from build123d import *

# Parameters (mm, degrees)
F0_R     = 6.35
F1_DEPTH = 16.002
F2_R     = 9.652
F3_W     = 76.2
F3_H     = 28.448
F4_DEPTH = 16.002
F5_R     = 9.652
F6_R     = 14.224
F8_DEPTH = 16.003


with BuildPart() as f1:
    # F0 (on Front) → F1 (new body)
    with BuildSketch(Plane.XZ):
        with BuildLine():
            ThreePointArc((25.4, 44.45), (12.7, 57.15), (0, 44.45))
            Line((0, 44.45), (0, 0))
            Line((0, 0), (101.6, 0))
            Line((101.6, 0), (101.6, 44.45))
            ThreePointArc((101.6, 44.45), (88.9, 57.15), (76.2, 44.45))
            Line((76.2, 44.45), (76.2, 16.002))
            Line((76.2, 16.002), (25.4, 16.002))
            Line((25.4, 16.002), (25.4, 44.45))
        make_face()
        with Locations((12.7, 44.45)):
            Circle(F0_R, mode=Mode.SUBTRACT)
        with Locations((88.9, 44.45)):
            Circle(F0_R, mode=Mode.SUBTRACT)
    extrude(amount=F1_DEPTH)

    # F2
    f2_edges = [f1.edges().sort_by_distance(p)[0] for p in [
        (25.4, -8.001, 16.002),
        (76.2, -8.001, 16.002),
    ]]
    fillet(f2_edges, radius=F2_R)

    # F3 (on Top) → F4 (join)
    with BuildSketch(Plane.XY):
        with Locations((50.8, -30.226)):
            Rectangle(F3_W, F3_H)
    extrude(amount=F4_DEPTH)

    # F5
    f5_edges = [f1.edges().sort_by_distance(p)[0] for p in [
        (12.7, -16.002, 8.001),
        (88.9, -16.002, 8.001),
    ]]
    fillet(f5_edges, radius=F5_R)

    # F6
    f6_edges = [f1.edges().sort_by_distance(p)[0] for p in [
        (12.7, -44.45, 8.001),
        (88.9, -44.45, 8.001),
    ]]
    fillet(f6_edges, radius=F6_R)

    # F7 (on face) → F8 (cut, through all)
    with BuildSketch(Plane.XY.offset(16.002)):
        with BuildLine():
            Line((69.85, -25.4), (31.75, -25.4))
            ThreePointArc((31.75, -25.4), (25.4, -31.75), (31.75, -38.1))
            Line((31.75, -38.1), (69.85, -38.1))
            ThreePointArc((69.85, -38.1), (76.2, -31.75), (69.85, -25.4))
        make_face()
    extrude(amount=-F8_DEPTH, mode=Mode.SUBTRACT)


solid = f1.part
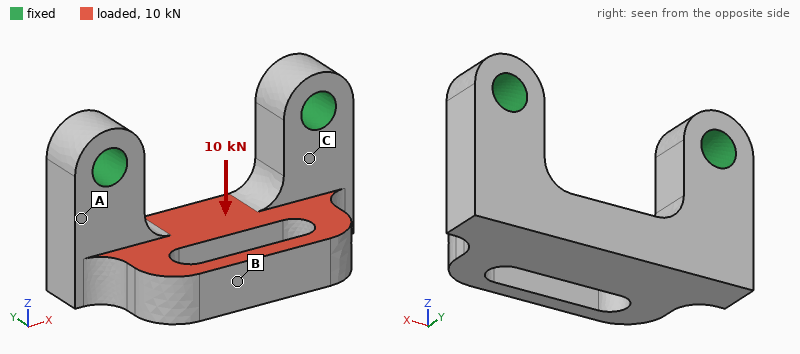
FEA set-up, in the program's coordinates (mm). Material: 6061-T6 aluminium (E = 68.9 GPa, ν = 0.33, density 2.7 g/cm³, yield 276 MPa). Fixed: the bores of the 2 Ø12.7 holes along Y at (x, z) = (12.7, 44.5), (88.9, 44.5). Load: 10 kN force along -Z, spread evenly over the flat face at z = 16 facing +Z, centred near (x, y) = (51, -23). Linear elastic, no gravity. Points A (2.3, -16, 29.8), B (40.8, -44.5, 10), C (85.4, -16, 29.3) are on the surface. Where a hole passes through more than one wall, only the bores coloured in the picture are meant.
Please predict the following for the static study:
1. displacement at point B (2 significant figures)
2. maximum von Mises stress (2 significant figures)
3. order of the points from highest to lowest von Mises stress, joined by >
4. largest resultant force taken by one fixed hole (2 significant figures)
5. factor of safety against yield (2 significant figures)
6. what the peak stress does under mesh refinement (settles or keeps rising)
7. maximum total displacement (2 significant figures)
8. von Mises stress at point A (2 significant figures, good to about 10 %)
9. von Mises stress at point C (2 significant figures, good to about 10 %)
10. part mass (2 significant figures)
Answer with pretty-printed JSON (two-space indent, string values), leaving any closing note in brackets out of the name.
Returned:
{
  "displacement at point B": "0.22 mm",
  "maximum von Mises stress": "150 MPa",
  "order of the points from highest to lowest von Mises stress, joined by >": "C > A > B",
  "largest resultant force taken by one fixed hole": "5.4 kN",
  "factor of safety against yield": "1.8",
  "what the peak stress does under mesh refinement": "settles",
  "maximum total displacement": "0.25 mm",
  "von Mises stress at point A": "61 MPa",
  "von Mises stress at point C": "93 MPa",
  "part mass": "210 g"
}
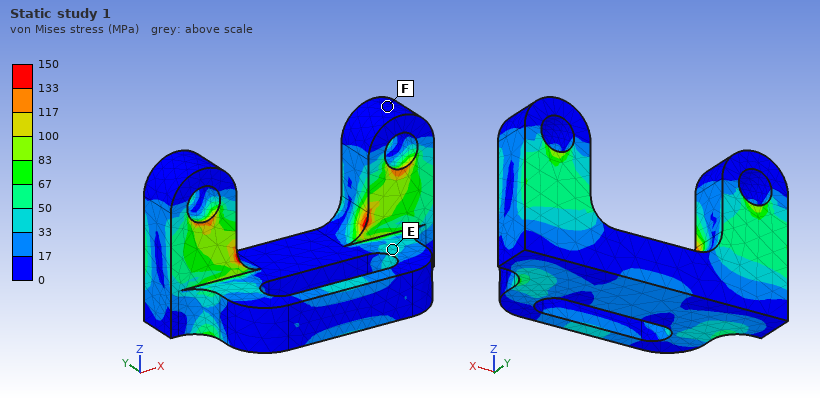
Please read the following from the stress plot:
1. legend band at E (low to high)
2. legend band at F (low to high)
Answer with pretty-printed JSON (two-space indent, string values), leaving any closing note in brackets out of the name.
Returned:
{
  "legend band at E": "33 to 50 MPa",
  "legend band at F": "0 to 17 MPa"
}
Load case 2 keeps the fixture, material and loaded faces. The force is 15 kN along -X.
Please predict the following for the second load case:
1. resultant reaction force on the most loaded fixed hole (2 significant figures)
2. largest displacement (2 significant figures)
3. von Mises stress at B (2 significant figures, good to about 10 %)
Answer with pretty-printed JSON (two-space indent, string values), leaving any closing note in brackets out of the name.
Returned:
{
  "resultant reaction force on the most loaded fixed hole": "8.1 kN",
  "largest displacement": "0.15 mm",
  "von Mises stress at B": "22 MPa"
}
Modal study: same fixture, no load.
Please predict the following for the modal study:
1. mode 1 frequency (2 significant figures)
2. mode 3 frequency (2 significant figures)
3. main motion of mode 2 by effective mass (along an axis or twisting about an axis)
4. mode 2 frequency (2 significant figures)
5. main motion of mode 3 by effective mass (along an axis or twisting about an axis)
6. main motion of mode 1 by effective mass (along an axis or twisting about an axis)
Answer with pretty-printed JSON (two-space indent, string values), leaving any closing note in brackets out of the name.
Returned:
{
  "mode 1 frequency": "3100 Hz",
  "mode 3 frequency": "7100 Hz",
  "main motion of mode 2 by effective mass": "along X",
  "mode 2 frequency": "5500 Hz",
  "main motion of mode 3 by effective mass": "along X",
  "main motion of mode 1 by effective mass": "along Y"
}
